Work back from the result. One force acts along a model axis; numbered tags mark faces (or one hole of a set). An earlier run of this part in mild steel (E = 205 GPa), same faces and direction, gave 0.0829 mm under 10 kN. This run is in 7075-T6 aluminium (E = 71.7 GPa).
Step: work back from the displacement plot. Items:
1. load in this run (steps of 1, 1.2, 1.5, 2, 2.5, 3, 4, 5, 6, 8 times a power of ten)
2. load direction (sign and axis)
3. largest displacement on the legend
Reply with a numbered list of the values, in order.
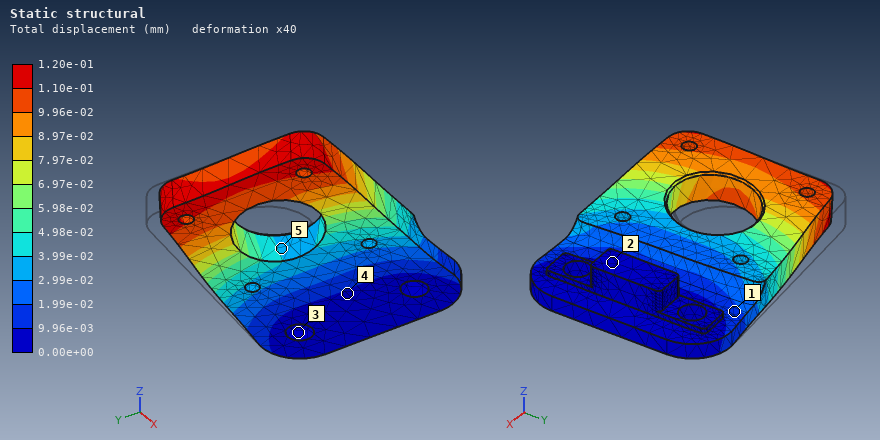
1. 5 kN
2. -Y
3. 1.20e-01 mm
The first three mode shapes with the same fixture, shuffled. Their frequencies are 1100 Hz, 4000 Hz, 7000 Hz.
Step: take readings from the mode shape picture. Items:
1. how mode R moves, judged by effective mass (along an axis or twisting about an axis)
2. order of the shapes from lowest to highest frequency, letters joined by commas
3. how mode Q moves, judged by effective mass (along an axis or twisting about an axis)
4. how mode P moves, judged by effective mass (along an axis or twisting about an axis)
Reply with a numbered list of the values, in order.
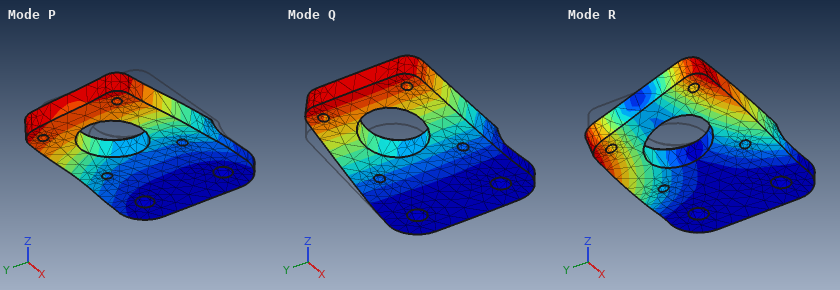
1. twisting about X
2. Q, R, P
3. along Z
4. along Y
